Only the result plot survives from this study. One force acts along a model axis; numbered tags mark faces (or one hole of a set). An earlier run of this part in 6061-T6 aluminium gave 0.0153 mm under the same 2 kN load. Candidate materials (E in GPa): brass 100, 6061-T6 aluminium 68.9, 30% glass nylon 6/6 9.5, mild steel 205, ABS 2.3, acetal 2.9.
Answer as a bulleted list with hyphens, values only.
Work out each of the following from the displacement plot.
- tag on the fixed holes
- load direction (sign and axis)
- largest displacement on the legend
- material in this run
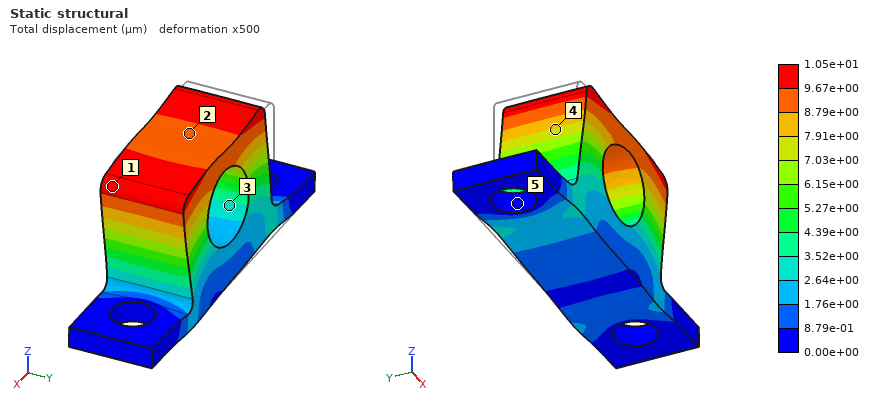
- 5
- +X
- 1.05e+01 µm
- brass
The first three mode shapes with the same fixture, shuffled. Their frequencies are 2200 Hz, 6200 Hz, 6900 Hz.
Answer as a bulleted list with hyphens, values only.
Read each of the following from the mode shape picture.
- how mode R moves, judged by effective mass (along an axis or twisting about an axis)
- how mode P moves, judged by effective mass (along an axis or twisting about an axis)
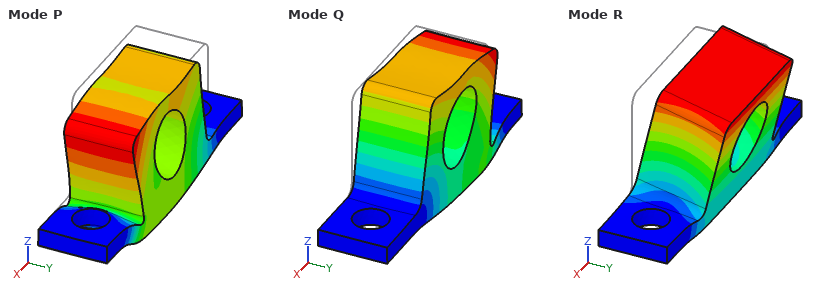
- along Y
- along Z
